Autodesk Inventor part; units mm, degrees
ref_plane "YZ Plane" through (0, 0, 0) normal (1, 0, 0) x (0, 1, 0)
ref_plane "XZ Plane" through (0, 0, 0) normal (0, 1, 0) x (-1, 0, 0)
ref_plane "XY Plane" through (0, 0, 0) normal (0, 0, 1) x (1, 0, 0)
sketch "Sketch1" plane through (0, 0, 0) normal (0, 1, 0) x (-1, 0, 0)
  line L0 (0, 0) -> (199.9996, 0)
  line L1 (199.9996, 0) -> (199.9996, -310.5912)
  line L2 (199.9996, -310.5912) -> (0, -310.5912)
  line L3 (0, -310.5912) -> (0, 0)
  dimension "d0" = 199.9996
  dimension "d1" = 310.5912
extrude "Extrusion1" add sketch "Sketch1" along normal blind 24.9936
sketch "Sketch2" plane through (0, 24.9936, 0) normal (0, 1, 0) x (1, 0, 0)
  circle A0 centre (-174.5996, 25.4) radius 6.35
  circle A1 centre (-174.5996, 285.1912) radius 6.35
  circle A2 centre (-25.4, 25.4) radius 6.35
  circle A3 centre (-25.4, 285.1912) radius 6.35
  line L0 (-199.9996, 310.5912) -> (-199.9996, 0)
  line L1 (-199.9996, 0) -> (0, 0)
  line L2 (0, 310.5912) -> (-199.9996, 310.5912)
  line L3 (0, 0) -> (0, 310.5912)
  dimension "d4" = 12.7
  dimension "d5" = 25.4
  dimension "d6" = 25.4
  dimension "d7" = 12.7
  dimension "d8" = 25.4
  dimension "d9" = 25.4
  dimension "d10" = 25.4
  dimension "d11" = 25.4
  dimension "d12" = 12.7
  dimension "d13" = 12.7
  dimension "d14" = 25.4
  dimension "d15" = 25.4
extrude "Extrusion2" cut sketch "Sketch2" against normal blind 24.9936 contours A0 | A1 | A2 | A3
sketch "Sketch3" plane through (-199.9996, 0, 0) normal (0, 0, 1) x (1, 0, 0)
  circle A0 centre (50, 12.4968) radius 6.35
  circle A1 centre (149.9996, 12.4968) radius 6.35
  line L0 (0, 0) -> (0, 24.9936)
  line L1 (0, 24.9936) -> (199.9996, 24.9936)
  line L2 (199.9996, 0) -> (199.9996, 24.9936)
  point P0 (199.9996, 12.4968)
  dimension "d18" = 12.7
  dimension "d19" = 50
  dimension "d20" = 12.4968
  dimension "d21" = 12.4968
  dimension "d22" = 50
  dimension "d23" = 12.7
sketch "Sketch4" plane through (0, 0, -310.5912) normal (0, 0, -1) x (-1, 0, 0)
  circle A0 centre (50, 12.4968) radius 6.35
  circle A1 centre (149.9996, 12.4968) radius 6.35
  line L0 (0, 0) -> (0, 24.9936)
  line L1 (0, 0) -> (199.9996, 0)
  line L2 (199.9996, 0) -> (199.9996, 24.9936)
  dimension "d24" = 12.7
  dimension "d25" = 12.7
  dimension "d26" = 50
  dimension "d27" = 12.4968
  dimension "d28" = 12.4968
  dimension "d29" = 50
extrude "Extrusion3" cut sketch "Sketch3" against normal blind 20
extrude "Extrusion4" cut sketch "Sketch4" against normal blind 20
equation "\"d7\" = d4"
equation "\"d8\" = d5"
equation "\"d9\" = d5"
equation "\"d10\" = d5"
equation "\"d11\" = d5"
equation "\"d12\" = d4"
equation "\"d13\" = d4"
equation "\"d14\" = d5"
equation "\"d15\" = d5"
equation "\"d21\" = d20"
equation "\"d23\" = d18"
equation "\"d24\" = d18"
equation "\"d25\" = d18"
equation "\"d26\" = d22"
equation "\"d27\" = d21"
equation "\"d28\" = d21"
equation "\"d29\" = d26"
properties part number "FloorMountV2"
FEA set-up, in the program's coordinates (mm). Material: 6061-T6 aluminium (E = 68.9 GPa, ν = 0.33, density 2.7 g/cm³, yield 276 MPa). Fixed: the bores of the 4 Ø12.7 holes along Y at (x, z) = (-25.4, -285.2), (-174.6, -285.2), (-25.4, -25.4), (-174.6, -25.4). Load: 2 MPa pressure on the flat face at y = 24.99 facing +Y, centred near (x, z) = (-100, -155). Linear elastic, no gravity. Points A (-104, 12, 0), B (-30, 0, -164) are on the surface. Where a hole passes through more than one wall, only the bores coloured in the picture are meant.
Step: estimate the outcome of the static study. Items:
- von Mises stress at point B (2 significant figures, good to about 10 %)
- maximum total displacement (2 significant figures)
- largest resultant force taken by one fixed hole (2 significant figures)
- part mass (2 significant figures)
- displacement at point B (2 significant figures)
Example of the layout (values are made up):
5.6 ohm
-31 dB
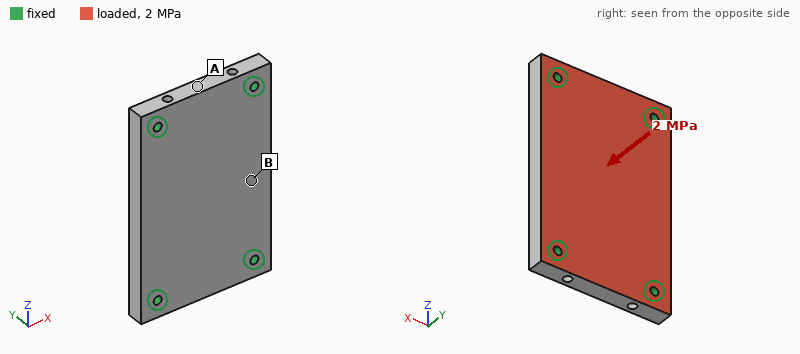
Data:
63 MPa
0.41 mm
31 kN
4.1 kg
0.39 mm
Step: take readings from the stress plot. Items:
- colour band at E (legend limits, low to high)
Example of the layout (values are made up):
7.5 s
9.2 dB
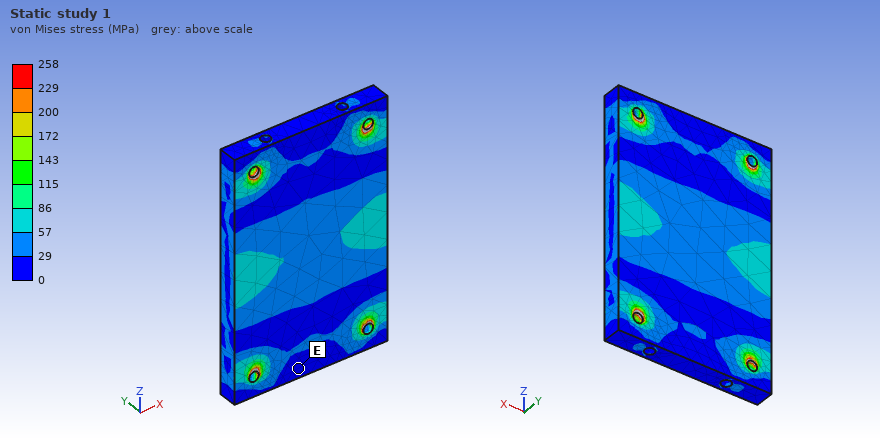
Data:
0 to 29 MPa
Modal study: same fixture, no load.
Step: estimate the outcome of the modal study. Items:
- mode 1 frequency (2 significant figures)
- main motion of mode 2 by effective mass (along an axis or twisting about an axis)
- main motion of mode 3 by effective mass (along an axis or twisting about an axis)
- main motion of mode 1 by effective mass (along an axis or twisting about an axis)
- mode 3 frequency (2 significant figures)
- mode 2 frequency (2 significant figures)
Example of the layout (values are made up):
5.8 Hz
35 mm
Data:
1500 Hz
twisting about Z
twisting about X
along Y
3800 Hz
2300 Hz
